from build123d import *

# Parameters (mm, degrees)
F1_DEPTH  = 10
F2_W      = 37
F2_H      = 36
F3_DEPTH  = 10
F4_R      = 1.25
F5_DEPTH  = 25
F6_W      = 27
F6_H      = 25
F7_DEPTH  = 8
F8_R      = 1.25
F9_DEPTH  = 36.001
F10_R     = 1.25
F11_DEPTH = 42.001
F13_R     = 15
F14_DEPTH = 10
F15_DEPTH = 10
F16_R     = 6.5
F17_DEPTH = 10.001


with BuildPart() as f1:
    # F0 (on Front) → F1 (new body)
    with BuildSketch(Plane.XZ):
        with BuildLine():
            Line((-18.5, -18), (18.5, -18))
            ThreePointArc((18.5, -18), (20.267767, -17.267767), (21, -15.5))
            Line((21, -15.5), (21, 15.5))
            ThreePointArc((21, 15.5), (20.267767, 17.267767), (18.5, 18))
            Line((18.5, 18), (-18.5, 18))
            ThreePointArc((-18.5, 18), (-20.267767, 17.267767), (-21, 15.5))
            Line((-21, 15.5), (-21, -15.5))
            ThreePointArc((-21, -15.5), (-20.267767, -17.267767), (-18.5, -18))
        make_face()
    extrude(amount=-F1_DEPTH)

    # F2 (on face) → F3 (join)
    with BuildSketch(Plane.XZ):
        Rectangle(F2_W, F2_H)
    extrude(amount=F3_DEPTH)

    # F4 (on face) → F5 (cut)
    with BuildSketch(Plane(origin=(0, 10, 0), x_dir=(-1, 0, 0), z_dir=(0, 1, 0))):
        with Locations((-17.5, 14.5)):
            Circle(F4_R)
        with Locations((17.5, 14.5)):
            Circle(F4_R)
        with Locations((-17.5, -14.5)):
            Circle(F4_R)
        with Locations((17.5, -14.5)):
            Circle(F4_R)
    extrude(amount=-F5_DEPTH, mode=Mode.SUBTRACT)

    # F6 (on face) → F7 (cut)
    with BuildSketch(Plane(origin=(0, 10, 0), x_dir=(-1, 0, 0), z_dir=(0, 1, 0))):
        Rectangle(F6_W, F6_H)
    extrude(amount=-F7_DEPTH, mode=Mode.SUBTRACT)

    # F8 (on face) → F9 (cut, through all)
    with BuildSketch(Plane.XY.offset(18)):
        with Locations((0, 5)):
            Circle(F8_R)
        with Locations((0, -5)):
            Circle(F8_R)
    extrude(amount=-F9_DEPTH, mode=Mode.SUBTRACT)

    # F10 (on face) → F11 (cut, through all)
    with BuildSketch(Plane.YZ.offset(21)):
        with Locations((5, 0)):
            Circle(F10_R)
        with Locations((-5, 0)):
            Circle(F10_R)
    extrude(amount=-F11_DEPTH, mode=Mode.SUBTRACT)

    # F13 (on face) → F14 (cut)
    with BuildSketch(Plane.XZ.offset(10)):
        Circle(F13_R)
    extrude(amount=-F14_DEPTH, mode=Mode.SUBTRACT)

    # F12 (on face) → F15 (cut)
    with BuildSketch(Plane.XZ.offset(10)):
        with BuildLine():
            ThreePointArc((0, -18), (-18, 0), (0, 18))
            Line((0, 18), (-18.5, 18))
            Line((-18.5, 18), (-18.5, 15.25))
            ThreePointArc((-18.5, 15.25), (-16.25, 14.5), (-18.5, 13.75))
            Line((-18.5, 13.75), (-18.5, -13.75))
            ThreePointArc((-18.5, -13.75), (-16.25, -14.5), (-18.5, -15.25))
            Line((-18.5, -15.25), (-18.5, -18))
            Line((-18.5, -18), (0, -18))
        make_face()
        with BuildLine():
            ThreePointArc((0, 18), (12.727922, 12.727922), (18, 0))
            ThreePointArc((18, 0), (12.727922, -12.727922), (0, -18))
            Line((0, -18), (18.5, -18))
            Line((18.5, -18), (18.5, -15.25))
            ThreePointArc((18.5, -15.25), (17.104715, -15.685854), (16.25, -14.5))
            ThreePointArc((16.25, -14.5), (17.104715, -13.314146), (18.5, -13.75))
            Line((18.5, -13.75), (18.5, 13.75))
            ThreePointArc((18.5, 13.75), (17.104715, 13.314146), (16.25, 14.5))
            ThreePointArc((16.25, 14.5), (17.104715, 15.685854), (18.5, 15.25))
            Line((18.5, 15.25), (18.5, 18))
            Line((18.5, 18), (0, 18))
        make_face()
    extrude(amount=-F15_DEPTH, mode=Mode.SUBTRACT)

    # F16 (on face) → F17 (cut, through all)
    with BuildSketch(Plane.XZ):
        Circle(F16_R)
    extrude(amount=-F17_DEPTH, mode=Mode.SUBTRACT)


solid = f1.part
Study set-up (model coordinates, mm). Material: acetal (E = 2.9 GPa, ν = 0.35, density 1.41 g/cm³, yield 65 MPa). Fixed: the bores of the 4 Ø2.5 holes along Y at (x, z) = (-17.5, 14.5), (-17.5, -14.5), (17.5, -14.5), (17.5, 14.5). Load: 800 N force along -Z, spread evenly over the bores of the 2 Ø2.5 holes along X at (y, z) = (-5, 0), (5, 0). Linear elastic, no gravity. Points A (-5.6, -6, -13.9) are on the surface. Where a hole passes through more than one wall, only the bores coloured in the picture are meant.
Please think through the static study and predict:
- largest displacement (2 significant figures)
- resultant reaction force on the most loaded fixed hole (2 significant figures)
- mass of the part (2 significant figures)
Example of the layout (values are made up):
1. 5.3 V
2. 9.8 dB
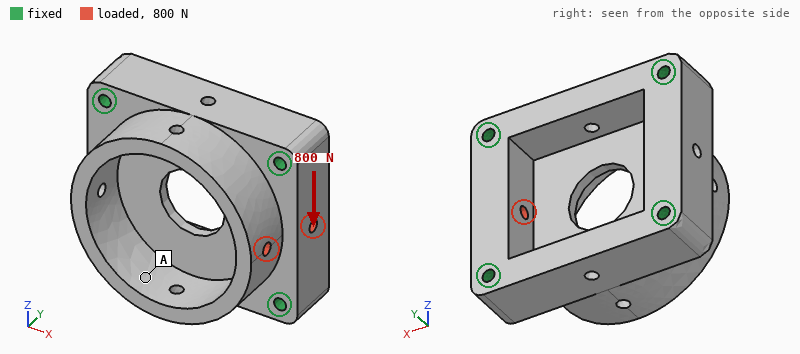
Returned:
1. 51 µm
2. 390 N
3. 17 g
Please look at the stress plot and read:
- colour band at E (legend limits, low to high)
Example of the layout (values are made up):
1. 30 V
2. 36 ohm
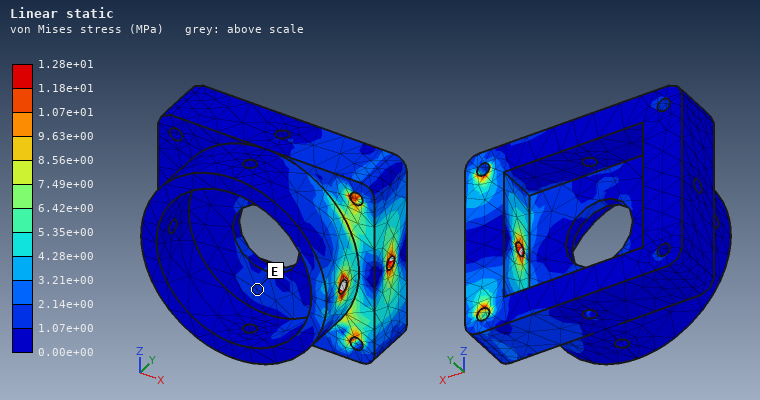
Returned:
1. 1.07e+00 to 2.14e+00 MPa
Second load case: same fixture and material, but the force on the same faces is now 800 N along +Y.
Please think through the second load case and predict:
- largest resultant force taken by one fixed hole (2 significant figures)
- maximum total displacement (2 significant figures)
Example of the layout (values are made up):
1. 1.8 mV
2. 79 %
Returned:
1. 410 N
2. 0.14 mm
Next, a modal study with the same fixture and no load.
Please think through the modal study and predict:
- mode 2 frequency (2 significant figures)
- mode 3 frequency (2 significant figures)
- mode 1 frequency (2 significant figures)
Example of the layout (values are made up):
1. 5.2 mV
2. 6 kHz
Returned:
1. 7100 Hz
2. 7200 Hz
3. 5900 Hz
